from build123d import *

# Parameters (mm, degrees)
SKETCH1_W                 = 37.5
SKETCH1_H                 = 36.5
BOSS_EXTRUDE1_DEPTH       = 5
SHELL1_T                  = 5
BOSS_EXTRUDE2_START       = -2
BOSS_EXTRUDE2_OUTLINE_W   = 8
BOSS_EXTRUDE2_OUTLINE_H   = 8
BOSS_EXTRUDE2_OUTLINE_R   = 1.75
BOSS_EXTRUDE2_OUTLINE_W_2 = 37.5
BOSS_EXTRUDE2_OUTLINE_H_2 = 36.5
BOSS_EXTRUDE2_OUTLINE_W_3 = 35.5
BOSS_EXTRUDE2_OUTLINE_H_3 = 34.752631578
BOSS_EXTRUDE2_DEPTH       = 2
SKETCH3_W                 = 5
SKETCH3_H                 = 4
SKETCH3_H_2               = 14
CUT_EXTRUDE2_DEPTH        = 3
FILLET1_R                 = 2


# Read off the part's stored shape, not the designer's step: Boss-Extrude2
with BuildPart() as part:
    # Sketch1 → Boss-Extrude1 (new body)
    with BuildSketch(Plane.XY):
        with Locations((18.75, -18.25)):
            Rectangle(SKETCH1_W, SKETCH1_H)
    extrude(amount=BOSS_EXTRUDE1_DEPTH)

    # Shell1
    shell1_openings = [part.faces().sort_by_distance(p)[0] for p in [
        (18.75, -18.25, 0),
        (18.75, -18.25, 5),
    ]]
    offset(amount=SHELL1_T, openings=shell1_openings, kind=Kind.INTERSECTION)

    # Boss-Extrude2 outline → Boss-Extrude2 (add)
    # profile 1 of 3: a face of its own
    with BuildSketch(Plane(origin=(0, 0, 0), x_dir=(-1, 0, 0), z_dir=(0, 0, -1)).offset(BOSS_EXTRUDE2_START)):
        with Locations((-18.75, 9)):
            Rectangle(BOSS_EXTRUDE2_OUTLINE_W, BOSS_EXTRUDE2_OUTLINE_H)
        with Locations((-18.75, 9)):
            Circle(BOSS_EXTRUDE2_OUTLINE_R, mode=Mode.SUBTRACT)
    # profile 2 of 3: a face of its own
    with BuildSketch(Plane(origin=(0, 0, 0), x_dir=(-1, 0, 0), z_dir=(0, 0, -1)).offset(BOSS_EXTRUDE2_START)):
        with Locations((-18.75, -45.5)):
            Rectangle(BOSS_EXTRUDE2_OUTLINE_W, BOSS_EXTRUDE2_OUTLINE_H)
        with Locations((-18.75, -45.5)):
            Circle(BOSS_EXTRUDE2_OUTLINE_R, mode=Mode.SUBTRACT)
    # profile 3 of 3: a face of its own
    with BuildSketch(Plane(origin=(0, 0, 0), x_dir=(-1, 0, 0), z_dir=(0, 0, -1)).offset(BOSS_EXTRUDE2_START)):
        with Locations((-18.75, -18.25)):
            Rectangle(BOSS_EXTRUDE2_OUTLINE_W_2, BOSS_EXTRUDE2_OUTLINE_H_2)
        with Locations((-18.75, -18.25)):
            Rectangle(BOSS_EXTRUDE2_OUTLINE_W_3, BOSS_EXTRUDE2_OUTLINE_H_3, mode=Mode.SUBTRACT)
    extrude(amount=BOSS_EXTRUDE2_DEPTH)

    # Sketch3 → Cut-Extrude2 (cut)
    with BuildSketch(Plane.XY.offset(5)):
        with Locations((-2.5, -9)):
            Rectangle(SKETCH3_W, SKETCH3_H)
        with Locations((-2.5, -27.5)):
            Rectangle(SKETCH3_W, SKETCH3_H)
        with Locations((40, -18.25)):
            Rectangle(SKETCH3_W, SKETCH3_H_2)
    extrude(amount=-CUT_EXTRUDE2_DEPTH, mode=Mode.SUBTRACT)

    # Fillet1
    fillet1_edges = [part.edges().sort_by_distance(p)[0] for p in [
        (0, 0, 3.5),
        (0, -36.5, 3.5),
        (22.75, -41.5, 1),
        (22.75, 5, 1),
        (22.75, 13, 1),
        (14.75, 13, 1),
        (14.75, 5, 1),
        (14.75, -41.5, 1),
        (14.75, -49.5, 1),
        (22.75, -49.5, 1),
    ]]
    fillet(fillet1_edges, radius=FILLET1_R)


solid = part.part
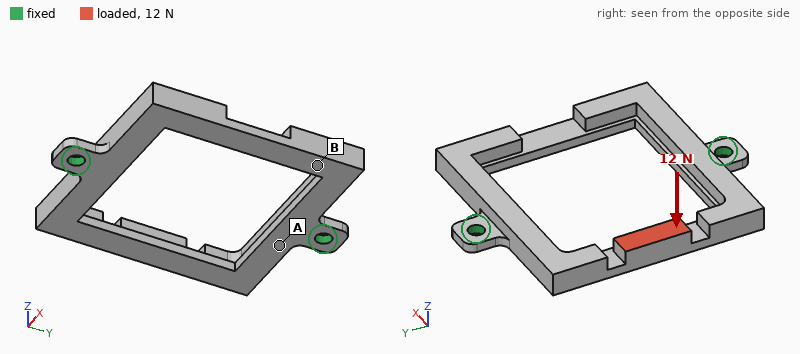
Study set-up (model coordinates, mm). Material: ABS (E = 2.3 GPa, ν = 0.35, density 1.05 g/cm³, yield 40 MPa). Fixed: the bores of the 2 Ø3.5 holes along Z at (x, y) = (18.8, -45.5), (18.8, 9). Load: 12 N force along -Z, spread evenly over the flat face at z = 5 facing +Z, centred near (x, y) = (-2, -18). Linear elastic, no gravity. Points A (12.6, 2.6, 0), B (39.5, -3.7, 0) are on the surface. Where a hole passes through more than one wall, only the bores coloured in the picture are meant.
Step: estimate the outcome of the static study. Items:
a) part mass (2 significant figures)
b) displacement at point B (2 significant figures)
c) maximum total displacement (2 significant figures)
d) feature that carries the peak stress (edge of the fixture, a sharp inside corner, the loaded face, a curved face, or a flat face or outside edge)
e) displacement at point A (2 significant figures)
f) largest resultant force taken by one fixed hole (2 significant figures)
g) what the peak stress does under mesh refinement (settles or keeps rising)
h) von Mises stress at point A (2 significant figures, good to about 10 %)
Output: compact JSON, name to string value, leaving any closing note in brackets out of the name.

{"part mass": "4.6 g", "displacement at point B": "0.25 mm", "maximum total displacement": "0.92 mm", "feature that carries the peak stress": "edge of the fixture", "displacement at point A": "0.17 mm", "largest resultant force taken by one fixed hole": "6.0 N", "what the peak stress does under mesh refinement": "keeps rising", "von Mises stress at point A": "4.5 MPa"}
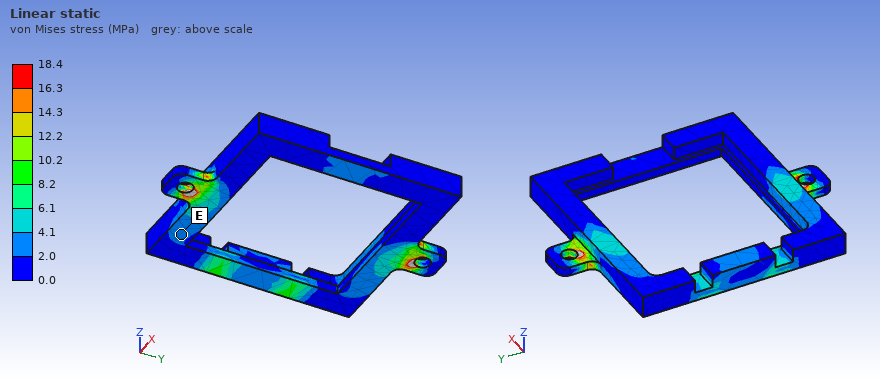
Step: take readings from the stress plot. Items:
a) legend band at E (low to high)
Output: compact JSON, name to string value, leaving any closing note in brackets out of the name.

{"legend band at E": "2.0 to 4.1 MPa"}
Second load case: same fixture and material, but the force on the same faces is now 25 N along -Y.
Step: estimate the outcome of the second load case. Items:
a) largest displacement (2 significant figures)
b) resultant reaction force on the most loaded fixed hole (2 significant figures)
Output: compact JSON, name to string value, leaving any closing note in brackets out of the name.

{"largest displacement": "0.23 mm", "resultant reaction force on the most loaded fixed hole": "14 N"}
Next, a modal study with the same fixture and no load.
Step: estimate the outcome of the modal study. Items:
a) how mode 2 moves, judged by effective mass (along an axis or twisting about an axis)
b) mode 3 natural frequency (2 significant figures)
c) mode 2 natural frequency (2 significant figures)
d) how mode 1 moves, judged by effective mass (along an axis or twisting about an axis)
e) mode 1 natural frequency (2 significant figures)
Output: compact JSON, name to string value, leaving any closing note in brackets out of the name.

{"how mode 2 moves, judged by effective mass": "along Z", "mode 3 natural frequency": "1000 Hz", "mode 2 natural frequency": "770 Hz", "how mode 1 moves, judged by effective mass": "twisting about Y", "mode 1 natural frequency": "490 Hz"}
